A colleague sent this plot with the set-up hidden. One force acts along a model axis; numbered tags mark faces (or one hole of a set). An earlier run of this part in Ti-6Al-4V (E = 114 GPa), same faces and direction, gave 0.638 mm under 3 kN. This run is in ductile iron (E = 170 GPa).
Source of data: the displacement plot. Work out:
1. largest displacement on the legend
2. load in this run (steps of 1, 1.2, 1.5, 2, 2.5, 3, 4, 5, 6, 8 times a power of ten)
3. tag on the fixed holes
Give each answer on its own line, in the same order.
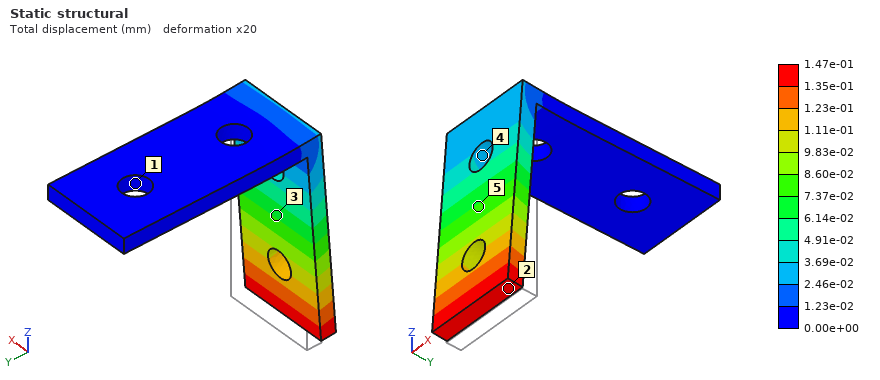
1.47e-01 mm
1 kN
1
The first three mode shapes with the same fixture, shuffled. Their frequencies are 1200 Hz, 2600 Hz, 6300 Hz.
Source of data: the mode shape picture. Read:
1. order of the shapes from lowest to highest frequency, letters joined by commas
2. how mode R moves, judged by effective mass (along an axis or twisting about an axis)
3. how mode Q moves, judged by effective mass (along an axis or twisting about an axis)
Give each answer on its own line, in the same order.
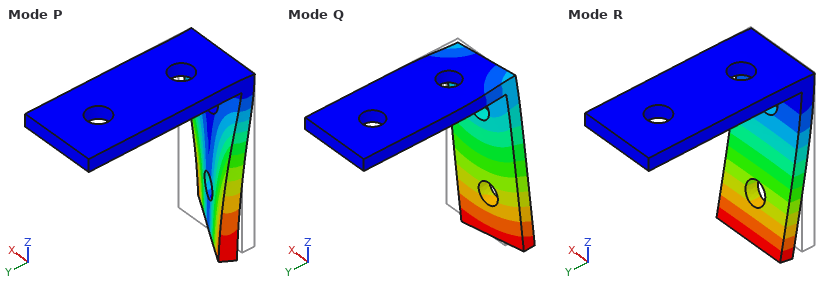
R, Q, P
along Y
along X
